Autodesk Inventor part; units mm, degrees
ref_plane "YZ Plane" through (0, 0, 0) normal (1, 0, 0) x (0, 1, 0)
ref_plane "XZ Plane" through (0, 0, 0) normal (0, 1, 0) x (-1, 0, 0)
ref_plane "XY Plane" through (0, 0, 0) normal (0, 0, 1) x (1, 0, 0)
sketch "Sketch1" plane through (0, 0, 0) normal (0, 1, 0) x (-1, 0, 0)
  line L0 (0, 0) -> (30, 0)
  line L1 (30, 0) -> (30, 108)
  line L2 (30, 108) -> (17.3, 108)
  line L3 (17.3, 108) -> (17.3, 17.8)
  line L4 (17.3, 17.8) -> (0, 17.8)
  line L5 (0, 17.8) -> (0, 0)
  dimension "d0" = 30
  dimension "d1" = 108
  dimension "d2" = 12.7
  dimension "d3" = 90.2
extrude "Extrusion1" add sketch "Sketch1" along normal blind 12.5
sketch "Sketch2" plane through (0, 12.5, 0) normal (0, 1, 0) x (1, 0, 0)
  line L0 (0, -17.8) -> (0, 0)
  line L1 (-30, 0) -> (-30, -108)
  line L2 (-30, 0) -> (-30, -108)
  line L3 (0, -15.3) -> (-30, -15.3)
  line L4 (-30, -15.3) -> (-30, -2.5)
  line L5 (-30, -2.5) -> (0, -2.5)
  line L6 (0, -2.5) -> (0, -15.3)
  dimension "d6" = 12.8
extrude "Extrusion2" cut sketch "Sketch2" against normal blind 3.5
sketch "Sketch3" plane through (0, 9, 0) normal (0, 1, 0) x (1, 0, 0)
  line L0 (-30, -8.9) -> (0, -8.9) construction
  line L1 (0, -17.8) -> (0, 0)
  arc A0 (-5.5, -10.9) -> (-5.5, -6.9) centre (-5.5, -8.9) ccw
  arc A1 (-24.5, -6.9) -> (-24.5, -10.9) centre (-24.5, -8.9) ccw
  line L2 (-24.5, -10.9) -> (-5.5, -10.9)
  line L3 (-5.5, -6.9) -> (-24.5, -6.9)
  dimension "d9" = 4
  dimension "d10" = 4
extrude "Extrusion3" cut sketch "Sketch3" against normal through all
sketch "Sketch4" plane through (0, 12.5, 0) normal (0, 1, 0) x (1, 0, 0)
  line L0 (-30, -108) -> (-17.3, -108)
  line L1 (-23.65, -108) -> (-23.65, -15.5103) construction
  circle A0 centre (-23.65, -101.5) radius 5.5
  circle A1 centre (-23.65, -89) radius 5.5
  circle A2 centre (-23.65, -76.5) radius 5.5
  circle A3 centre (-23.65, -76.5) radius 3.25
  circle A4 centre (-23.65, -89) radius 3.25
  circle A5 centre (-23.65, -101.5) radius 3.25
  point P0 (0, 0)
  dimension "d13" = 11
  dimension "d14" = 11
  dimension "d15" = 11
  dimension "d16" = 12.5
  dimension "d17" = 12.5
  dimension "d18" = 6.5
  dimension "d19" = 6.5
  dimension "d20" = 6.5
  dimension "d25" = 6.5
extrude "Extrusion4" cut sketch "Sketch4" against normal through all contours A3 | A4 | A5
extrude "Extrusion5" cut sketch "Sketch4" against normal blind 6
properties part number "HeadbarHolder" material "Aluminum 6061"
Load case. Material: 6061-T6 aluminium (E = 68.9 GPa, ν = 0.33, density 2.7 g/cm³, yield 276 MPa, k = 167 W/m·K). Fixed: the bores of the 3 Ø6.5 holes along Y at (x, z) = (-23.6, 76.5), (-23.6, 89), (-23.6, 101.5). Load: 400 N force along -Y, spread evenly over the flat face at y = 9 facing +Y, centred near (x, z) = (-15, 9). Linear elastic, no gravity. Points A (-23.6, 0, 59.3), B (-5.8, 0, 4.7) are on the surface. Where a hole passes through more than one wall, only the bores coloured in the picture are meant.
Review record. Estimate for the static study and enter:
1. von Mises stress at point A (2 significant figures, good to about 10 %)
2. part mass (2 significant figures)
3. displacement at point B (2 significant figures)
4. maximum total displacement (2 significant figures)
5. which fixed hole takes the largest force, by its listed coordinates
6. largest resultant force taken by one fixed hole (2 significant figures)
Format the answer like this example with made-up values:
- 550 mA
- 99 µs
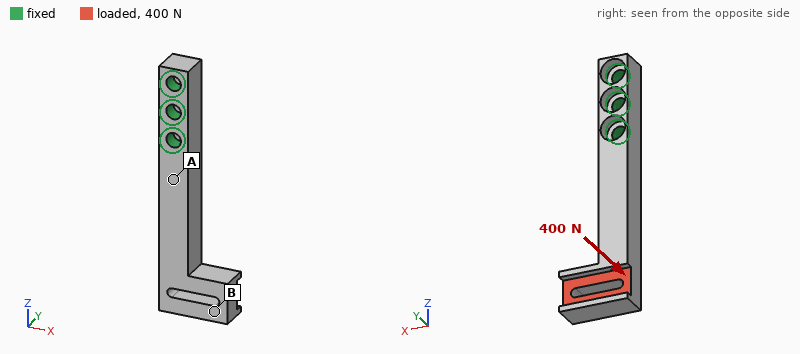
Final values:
- 64 MPa
- 45 g
- 0.54 mm
- 0.60 mm
- (-23.6, 76.5)
- 1.2 kN
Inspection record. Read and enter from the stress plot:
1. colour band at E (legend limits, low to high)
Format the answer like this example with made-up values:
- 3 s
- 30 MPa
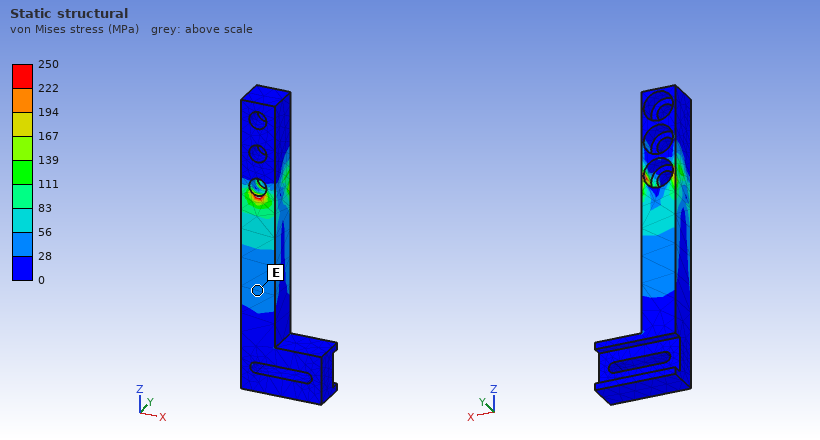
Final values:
- 28 to 56 MPa
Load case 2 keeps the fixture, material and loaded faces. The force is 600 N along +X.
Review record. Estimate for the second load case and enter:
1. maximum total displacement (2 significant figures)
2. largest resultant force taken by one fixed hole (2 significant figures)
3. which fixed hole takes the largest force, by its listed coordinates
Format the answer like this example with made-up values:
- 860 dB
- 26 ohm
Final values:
- 0.69 mm
- 1.4 kN
- (-23.6, 76.5)
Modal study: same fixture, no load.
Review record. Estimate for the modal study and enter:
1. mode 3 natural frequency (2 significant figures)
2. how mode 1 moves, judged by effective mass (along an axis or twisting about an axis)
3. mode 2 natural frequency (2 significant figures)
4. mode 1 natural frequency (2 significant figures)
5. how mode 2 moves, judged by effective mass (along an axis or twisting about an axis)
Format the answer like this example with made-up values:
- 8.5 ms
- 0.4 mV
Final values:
- 4400 Hz
- along Y
- 1300 Hz
- 1100 Hz
- along X
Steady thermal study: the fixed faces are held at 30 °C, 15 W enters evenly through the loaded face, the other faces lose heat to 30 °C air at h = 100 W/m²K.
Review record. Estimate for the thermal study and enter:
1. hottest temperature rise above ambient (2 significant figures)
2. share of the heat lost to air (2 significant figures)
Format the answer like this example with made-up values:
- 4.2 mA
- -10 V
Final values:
- 27 K
- 52 %
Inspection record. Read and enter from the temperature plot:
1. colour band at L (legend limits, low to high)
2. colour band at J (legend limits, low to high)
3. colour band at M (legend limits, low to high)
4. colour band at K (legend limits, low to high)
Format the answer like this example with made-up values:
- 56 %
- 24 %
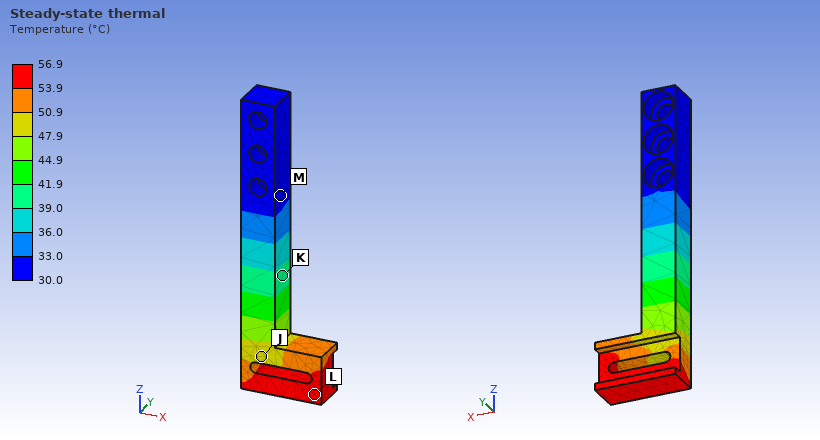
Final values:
- 53.9 to 56.9 °C
- 47.9 to 50.9 °C
- 30.0 to 33.0 °C
- 39.0 to 41.9 °C
